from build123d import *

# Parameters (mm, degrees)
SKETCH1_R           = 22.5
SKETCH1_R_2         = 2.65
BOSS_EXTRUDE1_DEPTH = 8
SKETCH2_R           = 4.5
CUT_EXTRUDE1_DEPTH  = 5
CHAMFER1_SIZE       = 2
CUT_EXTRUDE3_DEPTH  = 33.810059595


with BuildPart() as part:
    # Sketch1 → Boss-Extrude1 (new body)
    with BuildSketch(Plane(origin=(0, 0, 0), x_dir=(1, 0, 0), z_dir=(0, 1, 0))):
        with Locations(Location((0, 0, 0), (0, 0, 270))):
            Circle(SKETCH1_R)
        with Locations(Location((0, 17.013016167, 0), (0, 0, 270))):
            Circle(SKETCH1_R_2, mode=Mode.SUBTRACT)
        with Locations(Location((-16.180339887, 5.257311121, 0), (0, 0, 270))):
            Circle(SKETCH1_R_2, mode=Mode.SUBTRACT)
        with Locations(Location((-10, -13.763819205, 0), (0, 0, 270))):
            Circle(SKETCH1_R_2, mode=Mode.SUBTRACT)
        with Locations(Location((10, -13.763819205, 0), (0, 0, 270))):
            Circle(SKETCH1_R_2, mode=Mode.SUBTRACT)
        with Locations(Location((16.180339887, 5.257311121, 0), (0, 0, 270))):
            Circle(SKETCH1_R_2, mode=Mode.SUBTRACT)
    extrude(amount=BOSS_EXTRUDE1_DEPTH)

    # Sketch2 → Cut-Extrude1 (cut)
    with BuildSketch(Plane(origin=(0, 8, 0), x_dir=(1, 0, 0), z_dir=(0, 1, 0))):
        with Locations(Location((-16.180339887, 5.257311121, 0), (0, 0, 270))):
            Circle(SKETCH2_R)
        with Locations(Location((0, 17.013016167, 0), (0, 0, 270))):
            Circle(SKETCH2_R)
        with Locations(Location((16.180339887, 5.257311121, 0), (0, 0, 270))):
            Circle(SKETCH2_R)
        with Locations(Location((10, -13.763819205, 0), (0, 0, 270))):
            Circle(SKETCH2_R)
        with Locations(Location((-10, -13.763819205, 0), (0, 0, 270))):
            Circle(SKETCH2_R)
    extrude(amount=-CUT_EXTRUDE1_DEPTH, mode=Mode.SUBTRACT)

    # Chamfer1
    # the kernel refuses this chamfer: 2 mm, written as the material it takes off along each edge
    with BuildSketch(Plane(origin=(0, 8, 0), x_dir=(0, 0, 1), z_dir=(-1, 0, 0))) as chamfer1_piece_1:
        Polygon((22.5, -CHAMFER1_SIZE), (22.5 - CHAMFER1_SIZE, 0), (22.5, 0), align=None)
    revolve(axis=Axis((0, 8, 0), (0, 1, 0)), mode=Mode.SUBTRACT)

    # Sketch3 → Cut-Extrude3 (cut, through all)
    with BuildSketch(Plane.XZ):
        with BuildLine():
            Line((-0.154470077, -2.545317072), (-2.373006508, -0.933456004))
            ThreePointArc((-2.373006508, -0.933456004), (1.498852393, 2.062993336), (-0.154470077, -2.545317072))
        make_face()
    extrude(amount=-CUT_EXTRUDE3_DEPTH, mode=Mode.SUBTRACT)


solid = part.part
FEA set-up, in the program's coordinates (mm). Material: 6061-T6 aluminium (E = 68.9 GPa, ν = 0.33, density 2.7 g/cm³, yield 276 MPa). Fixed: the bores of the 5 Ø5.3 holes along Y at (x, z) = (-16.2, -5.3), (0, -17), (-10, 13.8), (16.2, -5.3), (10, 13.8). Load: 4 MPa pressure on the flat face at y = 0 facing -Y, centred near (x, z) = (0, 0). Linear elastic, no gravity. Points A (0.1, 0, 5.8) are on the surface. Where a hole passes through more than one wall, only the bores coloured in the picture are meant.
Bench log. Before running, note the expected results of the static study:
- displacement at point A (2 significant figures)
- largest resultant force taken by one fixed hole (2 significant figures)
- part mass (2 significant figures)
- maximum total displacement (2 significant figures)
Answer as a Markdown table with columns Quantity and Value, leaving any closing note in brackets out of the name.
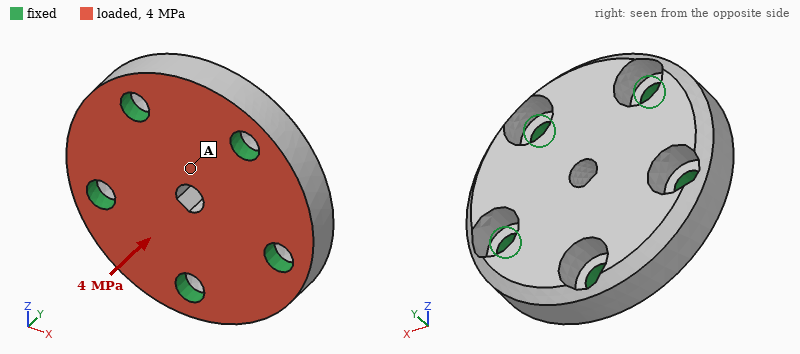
| Quantity | Value |
|---|---|
| displacement at point A | 5.0 µm |
| largest resultant force taken by one fixed hole | 1.2 kN |
| part mass | 28 g |
| maximum total displacement | 5.6 µm |
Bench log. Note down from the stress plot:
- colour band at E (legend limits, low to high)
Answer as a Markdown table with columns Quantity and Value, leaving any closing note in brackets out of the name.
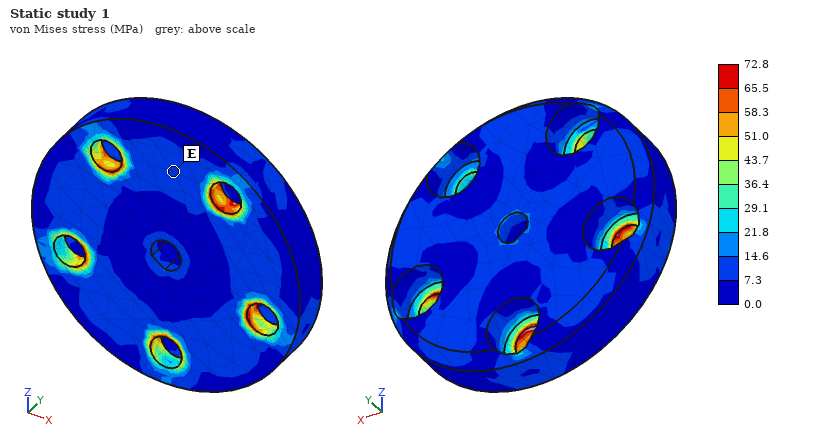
| Quantity | Value |
|---|---|
| colour band at E | 7.3 to 14.6 MPa |
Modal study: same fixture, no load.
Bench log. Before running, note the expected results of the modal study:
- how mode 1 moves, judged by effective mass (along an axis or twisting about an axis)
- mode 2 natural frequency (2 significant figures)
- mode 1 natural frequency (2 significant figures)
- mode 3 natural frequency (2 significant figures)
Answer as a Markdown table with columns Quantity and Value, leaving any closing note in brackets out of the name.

| Quantity | Value |
|---|---|
| how mode 1 moves, judged by effective mass | along Y |
| mode 2 natural frequency | 37 kHz |
| mode 1 natural frequency | 34 kHz |
| mode 3 natural frequency | 37 kHz |
